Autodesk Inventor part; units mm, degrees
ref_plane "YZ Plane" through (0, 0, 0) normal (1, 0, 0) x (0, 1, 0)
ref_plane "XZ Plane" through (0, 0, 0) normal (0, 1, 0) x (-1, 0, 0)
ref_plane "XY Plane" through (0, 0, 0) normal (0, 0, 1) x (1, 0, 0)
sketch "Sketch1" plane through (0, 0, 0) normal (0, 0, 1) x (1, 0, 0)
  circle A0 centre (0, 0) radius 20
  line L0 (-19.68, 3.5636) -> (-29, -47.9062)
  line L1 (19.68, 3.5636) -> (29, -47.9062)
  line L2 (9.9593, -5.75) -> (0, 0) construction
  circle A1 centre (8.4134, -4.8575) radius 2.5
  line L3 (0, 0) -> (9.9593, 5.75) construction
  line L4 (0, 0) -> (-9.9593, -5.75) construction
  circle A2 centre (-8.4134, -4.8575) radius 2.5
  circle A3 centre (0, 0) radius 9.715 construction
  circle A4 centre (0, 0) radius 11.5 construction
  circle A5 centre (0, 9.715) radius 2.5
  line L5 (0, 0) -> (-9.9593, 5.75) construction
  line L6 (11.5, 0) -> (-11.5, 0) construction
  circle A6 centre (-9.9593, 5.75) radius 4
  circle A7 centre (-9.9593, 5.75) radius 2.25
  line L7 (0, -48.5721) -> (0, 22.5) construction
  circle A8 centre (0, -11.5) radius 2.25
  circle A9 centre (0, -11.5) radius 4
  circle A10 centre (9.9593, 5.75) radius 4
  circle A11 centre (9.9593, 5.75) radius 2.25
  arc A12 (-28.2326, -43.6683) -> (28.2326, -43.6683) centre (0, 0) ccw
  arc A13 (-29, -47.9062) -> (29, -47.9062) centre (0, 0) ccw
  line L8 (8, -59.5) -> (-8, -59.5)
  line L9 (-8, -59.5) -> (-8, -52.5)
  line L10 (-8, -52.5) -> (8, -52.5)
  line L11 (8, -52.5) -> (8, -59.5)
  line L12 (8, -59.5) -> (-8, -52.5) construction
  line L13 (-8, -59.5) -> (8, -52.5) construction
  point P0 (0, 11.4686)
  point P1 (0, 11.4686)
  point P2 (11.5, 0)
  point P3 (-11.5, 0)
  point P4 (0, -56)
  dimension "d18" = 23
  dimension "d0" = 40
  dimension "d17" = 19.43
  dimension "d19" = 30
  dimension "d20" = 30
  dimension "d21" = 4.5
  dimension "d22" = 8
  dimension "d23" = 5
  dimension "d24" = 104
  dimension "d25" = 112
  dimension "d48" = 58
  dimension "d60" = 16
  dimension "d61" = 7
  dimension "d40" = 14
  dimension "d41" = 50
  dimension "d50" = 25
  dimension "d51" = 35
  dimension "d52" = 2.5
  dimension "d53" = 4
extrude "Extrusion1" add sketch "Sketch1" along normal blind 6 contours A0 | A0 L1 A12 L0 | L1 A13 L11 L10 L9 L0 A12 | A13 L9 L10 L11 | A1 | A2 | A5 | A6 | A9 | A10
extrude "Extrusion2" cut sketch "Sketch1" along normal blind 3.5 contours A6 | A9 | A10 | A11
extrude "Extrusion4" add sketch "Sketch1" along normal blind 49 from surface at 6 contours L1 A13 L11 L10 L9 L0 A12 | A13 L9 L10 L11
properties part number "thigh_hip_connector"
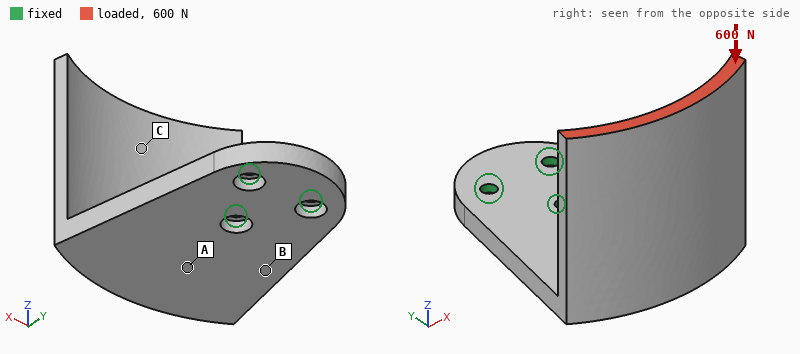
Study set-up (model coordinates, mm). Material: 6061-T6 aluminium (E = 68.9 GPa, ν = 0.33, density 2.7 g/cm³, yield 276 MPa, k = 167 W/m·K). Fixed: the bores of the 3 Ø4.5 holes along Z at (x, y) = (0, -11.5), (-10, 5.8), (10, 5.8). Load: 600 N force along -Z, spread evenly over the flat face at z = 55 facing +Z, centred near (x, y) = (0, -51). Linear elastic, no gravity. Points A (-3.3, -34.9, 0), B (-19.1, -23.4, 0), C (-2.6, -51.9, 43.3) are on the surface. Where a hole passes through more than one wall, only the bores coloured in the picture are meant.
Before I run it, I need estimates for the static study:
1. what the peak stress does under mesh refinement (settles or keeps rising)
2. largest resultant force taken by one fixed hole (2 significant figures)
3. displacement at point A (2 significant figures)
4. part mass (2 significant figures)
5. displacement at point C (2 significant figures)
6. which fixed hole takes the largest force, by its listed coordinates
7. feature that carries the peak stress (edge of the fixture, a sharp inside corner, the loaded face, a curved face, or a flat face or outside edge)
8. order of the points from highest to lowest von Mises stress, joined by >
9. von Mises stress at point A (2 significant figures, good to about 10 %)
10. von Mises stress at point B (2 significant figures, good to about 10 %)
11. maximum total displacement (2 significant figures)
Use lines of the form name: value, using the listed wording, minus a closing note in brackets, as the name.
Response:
what the peak stress does under mesh refinement: keeps rising
largest resultant force taken by one fixed hole: 2.2 kN
displacement at point A: 0.16 mm
part mass: 84 g
displacement at point C: 0.51 mm
which fixed hole takes the largest force, by its listed coordinates: (0, -11.5)
feature that carries the peak stress: edge of the fixture
order of the points from highest to lowest von Mises stress, joined by >: B > A > C
von Mises stress at point A: 26 MPa
von Mises stress at point B: 55 MPa
maximum total displacement: 0.63 mm
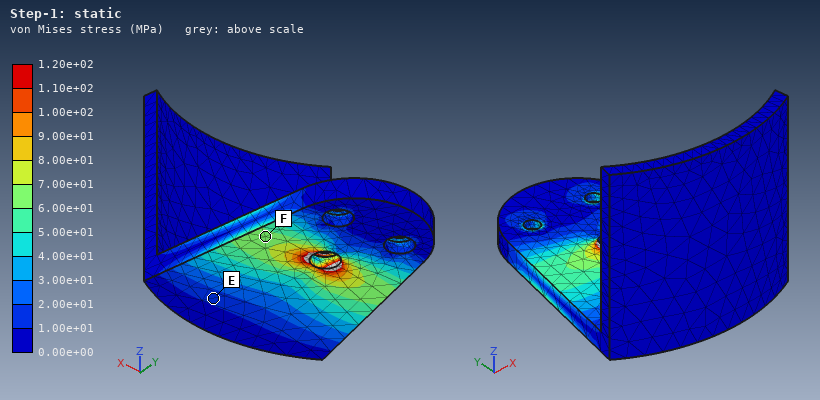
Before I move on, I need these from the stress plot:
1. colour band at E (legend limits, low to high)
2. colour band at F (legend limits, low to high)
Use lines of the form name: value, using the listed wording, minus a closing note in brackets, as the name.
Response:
colour band at E: 1.00e+01 to 2.00e+01 MPa
colour band at F: 6.00e+01 to 7.00e+01 MPa
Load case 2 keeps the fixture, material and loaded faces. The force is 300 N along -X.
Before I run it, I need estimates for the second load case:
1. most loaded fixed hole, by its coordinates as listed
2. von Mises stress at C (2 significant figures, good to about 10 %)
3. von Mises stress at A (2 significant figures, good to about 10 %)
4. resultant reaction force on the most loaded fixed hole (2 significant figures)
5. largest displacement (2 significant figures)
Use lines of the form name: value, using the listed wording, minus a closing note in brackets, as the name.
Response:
most loaded fixed hole, by its coordinates as listed: (0, -11.5)
von Mises stress at C: 14 MPa
von Mises stress at A: 36 MPa
resultant reaction force on the most loaded fixed hole: 1.2 kN
largest displacement: 0.52 mm
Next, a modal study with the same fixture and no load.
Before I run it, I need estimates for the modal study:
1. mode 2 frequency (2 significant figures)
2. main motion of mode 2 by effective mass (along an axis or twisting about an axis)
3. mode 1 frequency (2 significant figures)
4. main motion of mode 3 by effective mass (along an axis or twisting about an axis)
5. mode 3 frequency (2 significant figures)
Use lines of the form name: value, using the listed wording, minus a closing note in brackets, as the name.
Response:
mode 2 frequency: 1000 Hz
main motion of mode 2 by effective mass: along X
mode 1 frequency: 750 Hz
main motion of mode 3 by effective mass: along Z
mode 3 frequency: 1800 Hz
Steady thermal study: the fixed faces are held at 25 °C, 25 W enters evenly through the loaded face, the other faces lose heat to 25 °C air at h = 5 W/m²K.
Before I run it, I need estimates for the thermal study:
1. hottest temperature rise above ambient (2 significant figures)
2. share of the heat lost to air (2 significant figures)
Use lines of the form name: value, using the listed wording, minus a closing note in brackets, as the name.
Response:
hottest temperature rise above ambient: 54 K
share of the heat lost to air: 6.7 %
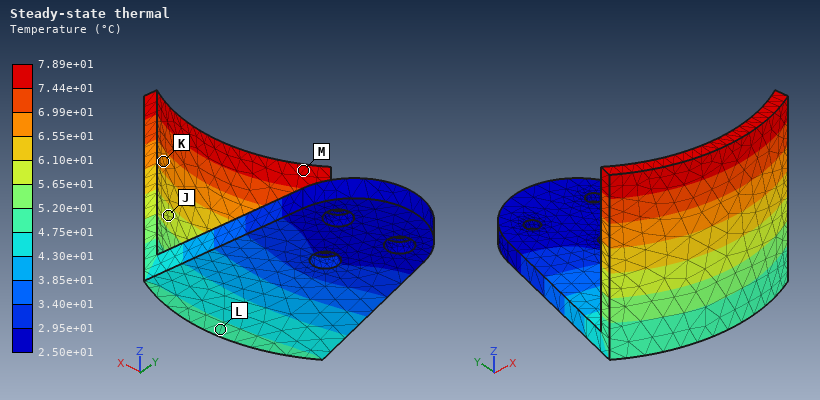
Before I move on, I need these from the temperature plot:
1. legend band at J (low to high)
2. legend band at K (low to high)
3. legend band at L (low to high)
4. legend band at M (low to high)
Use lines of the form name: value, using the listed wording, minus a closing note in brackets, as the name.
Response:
legend band at J: 5.65e+01 to 6.10e+01 °C
legend band at K: 6.55e+01 to 6.99e+01 °C
legend band at L: 4.75e+01 to 5.20e+01 °C
legend band at M: 7.44e+01 to 7.89e+01 °C
